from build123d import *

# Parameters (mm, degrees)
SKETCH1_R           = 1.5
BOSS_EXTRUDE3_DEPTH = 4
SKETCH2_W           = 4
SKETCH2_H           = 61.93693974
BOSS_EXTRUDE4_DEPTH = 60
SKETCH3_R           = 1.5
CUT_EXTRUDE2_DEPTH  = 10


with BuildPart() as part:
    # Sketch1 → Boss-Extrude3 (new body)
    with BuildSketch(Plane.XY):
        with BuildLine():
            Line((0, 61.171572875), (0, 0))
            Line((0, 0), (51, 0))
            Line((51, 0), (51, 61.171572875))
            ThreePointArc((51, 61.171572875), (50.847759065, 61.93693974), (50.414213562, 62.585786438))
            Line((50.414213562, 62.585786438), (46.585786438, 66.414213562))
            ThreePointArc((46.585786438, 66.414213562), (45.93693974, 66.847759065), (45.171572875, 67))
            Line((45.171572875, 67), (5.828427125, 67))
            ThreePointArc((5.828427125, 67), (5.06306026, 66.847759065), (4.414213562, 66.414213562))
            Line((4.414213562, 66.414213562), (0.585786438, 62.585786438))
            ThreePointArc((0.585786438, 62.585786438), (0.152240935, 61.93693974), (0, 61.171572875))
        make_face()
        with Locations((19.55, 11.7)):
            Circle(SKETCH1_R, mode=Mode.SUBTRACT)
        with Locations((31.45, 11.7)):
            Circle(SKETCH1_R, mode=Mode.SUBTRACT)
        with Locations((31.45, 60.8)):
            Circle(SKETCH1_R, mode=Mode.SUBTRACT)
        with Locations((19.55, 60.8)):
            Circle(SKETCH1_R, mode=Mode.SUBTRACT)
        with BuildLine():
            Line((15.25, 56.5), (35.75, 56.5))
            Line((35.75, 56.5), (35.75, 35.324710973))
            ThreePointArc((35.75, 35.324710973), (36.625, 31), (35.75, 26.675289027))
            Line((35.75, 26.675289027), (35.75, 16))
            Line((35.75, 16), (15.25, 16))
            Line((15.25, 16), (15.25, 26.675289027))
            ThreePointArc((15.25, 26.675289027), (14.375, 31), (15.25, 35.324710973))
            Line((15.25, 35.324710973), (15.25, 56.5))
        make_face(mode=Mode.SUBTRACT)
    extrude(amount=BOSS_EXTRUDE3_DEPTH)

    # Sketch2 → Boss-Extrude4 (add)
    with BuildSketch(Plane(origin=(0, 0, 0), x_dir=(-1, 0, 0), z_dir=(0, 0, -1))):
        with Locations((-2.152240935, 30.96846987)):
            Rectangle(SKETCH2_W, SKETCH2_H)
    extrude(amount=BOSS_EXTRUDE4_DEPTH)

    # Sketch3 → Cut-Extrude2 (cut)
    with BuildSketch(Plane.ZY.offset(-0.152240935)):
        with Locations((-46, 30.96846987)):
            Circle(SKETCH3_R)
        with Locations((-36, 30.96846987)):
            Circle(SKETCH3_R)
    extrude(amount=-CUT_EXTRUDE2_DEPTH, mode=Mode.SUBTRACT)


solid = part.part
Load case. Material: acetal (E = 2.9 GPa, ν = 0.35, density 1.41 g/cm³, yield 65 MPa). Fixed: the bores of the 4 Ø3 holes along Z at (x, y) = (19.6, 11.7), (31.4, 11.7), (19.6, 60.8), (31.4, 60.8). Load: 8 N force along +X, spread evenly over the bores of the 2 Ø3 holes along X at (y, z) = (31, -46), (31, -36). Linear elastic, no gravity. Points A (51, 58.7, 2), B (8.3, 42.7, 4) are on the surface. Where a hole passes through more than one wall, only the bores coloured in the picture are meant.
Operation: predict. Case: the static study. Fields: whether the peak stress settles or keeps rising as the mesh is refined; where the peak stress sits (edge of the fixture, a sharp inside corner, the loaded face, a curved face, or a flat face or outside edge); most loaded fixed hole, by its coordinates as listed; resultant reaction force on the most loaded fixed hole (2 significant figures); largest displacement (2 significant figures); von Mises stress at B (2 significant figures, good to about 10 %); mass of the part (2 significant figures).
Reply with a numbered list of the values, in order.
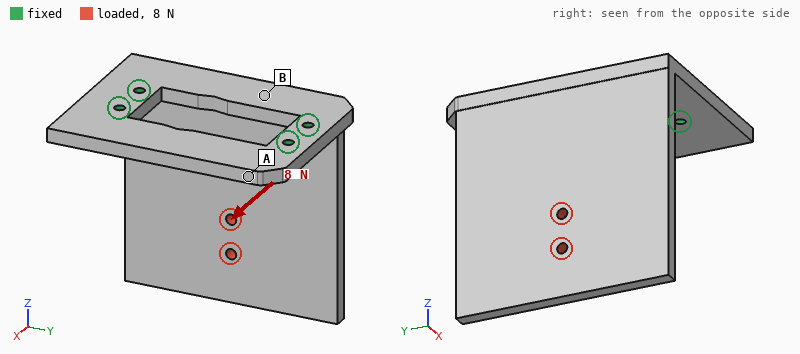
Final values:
1. keeps rising
2. edge of the fixture
3. (19.6, 11.7)
4. 7.9 N
5. 1.1 mm
6. 1.1 MPa
7. 35 g
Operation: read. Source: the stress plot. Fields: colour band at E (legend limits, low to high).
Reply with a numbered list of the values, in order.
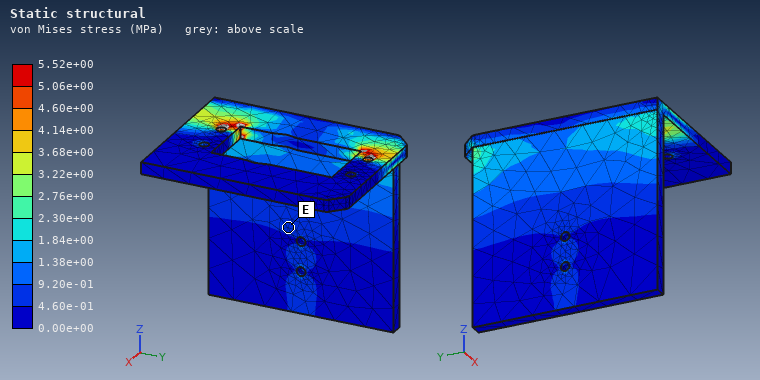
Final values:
1. 4.60e-01 to 9.20e-01 MPa
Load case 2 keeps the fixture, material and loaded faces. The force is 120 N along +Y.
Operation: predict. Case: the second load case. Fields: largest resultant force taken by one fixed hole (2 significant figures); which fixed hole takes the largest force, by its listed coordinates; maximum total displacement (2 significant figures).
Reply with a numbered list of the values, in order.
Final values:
1. 150 N
2. (19.6, 11.7)
3. 1.2 mm
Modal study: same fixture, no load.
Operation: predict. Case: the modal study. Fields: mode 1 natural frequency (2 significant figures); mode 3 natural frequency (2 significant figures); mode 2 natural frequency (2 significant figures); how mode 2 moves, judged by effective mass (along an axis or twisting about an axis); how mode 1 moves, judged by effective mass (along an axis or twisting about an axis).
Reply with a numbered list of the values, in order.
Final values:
1. 140 Hz
2. 620 Hz
3. 430 Hz
4. along Y
5. along X
